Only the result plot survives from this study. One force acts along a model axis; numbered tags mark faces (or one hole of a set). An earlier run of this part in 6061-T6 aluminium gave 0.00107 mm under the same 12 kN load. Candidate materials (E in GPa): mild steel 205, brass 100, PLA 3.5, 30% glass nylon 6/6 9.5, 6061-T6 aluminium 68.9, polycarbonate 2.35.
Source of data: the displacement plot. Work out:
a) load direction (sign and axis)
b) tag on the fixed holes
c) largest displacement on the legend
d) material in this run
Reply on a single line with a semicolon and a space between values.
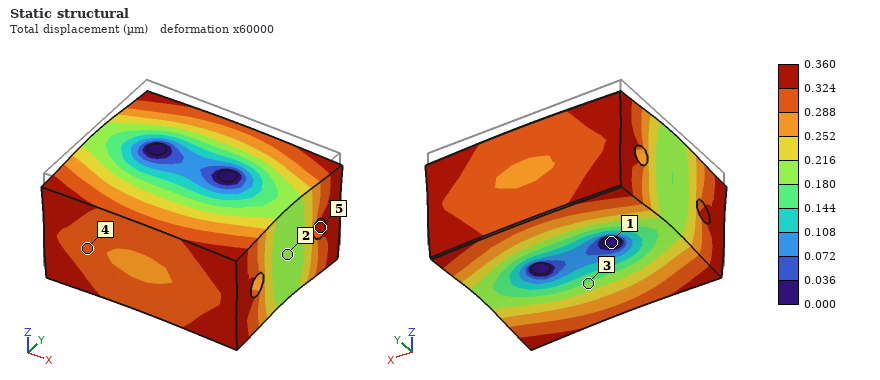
-Z; 1; 0.360 µm; mild steel
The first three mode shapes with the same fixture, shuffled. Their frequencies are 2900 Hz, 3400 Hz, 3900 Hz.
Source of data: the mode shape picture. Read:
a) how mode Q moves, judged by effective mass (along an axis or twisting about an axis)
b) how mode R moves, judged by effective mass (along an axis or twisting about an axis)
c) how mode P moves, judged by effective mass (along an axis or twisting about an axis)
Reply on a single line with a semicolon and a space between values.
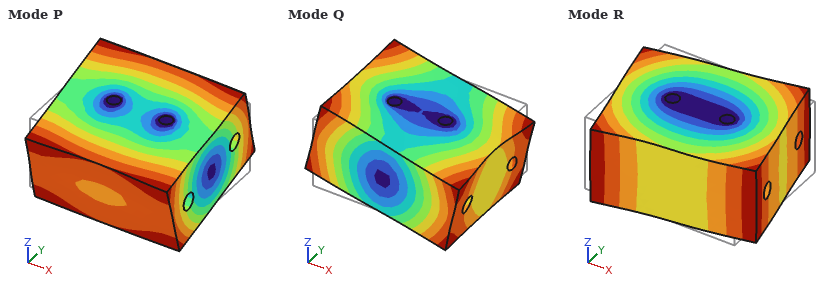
twisting about Y; twisting about Z; twisting about X
